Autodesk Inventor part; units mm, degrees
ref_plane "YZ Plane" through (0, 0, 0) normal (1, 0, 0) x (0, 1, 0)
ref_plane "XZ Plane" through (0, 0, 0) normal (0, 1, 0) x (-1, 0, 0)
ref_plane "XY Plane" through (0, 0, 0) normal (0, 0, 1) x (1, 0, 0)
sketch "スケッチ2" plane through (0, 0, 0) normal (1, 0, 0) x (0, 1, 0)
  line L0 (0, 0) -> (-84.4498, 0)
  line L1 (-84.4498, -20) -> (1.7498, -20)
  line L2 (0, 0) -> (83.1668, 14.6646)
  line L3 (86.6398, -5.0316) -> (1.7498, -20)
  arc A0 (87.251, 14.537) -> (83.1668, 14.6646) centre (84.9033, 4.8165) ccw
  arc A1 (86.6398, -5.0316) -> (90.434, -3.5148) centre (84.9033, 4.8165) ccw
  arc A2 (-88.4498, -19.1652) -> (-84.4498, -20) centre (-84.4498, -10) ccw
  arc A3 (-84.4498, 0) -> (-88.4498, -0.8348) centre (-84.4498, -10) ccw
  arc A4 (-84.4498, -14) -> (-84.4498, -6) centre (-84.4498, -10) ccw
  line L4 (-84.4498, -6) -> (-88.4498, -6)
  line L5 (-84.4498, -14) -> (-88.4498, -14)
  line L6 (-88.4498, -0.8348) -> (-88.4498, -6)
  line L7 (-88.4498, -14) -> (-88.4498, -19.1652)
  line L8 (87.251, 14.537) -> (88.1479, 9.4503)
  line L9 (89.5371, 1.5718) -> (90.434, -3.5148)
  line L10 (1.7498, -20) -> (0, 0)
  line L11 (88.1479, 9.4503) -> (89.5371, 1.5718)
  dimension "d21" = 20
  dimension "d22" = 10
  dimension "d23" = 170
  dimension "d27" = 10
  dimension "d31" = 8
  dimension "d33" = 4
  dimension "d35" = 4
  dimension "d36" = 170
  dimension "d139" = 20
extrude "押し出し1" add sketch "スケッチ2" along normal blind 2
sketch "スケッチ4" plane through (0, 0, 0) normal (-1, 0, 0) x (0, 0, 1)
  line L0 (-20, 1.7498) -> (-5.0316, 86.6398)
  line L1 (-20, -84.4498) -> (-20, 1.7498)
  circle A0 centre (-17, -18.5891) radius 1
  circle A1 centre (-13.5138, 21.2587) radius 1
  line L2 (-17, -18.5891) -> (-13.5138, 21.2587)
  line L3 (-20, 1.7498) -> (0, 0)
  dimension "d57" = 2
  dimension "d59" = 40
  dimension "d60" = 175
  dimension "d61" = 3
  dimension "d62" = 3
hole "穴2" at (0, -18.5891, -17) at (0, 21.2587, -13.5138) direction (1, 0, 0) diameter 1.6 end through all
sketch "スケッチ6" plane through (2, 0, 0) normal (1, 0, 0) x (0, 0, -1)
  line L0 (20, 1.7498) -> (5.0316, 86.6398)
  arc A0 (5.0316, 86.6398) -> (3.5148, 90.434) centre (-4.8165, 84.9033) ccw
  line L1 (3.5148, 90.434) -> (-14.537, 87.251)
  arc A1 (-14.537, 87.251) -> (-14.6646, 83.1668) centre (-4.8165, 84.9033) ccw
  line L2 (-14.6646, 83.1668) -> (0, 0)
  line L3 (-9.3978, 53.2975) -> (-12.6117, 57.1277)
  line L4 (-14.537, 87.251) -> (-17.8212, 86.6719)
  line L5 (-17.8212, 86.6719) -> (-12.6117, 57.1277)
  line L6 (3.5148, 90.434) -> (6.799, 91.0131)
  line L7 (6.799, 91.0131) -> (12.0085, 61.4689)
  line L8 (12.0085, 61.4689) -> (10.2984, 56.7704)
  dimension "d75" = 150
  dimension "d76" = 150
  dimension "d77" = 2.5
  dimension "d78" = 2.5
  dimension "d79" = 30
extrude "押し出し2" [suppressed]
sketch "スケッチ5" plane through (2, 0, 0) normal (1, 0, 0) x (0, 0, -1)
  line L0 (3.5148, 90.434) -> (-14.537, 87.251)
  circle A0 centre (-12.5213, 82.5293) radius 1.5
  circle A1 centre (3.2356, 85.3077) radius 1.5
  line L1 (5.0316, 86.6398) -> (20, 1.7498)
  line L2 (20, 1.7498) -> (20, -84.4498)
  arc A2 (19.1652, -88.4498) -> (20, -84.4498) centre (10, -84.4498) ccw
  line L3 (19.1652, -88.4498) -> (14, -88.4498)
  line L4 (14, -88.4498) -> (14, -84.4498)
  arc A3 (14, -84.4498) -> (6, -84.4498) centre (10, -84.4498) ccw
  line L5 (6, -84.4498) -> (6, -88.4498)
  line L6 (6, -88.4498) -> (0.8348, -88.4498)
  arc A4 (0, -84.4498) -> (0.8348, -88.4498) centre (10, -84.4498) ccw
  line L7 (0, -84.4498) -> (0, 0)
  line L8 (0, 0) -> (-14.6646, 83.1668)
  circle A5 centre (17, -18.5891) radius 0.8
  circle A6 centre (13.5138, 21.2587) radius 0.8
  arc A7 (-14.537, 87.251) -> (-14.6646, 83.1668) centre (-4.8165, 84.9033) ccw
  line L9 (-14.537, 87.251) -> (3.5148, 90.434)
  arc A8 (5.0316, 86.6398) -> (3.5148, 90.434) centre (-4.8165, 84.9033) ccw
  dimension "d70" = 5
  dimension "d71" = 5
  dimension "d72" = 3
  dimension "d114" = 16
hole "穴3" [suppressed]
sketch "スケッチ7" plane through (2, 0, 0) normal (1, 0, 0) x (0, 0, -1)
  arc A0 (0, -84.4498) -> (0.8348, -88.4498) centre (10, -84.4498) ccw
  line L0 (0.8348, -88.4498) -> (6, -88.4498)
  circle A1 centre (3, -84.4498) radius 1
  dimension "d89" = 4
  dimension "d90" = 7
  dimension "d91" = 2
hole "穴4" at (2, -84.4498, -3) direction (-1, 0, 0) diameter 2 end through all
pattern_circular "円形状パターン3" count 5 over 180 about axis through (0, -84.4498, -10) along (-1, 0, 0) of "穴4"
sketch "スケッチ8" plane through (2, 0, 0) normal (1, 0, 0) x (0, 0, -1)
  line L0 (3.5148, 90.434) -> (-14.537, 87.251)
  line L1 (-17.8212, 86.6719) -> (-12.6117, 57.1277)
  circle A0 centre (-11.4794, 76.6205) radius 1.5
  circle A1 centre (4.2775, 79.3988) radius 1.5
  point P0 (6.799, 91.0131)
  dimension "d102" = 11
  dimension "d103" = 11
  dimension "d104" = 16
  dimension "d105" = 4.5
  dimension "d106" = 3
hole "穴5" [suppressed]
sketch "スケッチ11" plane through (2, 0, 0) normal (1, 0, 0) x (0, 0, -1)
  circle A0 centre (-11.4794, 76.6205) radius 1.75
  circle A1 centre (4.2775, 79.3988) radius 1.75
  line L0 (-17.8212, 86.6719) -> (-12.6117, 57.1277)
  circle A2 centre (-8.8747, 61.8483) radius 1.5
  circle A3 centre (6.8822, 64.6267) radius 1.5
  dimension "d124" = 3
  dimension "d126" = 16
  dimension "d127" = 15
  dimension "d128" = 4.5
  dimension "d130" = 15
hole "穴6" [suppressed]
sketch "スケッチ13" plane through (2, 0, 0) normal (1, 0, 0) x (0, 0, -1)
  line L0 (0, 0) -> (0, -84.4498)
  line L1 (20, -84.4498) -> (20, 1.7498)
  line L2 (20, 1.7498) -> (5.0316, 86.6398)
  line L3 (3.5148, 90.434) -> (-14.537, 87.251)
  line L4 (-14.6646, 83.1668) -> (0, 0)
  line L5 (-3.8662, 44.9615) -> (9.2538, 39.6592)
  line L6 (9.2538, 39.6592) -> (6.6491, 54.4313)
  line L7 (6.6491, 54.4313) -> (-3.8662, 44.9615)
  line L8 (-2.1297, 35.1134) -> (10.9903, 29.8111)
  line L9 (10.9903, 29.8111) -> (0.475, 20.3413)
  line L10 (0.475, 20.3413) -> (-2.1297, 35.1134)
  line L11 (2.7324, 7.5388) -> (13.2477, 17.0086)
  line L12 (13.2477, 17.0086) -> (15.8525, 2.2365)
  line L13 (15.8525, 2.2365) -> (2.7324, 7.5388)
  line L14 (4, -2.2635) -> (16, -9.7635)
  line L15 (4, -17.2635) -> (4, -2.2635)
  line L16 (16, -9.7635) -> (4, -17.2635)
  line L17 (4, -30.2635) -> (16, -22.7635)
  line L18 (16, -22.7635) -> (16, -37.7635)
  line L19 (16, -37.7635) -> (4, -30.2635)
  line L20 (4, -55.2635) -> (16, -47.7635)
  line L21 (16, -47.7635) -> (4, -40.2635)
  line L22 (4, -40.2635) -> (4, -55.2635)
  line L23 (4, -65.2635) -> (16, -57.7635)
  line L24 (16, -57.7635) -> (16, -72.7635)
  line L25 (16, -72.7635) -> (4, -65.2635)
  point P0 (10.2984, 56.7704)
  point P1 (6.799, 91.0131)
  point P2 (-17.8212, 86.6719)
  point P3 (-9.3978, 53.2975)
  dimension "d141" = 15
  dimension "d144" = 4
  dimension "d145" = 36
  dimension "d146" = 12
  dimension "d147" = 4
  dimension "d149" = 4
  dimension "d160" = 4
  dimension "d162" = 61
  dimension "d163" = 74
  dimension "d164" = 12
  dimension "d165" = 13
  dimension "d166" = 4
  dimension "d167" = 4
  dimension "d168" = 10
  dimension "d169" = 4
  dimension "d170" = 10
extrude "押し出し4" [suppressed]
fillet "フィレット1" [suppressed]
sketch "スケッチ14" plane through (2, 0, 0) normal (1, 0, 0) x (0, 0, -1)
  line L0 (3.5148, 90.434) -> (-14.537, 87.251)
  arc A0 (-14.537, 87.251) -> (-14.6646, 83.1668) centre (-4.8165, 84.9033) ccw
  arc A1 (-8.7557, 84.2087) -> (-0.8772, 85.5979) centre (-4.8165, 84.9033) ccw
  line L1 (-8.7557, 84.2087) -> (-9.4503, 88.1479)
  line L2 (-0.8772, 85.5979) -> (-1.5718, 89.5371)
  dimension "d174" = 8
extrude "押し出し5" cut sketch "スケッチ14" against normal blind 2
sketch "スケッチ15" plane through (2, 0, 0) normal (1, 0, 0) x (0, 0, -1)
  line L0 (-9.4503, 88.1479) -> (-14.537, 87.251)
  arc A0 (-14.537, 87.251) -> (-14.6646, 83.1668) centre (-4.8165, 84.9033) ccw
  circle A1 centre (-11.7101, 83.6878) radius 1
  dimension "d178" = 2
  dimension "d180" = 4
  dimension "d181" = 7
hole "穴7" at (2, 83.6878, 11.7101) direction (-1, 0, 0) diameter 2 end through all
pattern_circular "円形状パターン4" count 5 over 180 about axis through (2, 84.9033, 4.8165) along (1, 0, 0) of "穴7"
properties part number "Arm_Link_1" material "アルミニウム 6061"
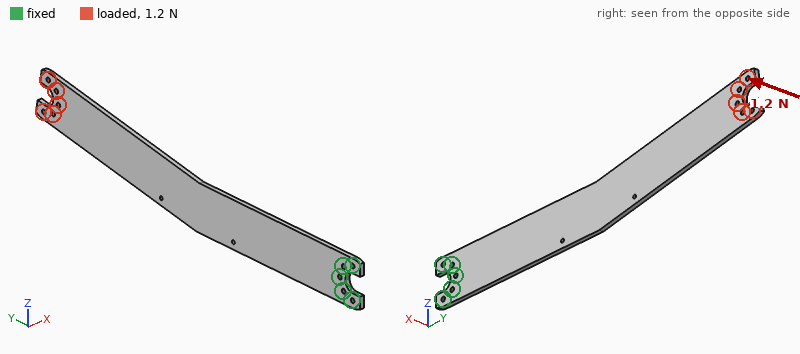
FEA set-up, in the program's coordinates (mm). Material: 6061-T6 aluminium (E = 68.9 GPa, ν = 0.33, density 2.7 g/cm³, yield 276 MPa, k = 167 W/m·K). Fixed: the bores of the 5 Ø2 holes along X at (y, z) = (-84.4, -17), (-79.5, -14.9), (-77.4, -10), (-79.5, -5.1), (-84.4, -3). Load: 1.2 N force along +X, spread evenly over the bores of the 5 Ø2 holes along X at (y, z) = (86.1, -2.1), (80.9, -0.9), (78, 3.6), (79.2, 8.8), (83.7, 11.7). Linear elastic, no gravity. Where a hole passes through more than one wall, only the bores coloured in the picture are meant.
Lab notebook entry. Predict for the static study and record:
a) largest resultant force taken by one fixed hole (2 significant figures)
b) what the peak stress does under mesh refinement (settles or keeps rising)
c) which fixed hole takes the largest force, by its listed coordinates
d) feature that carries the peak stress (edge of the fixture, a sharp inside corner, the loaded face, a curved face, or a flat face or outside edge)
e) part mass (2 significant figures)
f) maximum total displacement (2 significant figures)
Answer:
19 N
keeps rising
(-77.4, -10)
edge of the fixture
18 g
1.9 mm
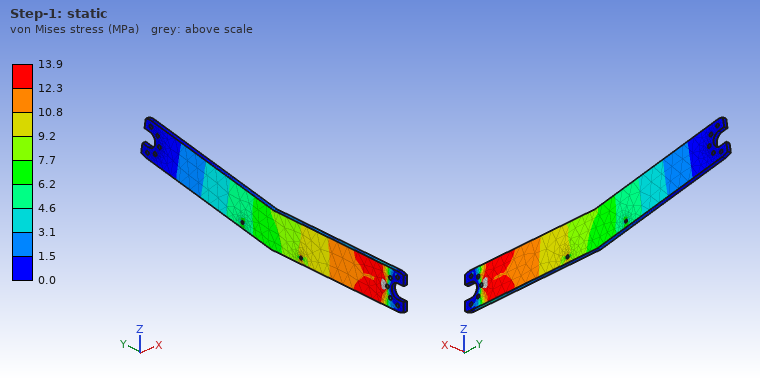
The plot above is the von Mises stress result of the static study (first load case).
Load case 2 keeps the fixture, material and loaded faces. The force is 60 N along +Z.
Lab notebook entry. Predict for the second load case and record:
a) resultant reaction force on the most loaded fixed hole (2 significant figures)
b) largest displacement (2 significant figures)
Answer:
500 N
1.0 mm
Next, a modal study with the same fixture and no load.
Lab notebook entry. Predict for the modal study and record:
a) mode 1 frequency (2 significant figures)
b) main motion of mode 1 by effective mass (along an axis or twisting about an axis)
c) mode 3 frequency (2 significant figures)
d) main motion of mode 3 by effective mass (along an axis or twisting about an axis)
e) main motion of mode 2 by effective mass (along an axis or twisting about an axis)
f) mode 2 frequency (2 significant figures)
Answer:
61 Hz
along X
570 Hz
along Z
along X
370 Hz
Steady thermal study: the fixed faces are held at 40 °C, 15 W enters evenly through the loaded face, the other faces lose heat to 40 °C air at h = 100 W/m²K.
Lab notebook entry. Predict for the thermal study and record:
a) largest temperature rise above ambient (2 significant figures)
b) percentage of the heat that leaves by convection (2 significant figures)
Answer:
80 K
97 %
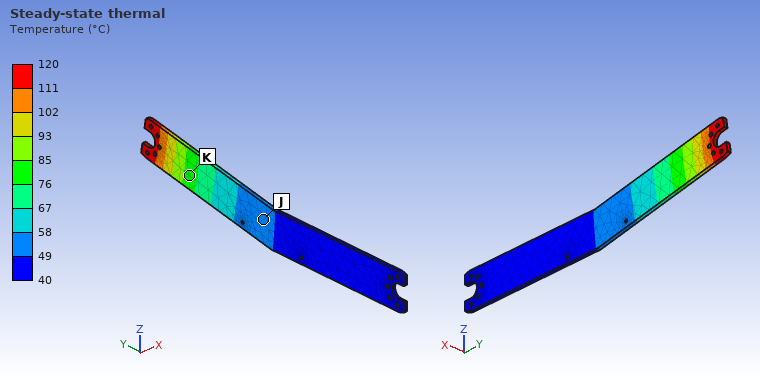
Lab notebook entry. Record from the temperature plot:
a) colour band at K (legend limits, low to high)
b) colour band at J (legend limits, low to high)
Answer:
76 to 85 °C
49 to 58 °C
